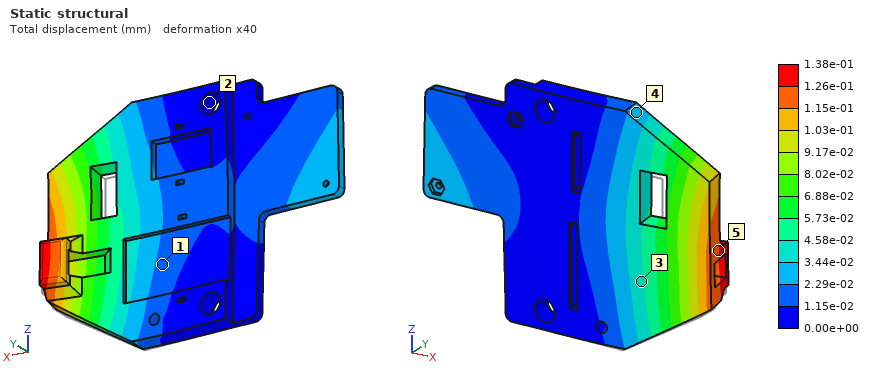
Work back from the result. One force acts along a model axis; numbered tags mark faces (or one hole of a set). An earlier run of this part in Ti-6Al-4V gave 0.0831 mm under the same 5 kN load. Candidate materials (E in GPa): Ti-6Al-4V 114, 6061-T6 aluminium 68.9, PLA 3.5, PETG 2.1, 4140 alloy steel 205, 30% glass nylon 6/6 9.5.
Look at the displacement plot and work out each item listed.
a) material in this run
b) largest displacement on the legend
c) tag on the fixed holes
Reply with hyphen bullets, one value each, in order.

- 6061-T6 aluminium
- 1.38e-01 mm
- 2
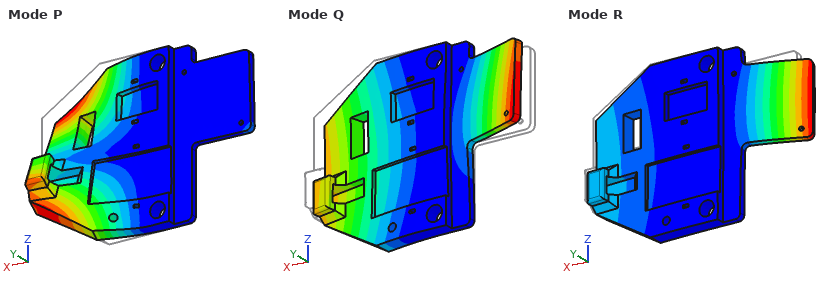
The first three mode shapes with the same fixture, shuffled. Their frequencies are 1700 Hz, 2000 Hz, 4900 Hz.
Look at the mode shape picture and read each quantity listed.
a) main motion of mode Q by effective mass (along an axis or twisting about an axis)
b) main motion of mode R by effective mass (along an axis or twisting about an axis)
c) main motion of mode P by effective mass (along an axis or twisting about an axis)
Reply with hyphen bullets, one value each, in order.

- along Y
- along Y
- twisting about X
